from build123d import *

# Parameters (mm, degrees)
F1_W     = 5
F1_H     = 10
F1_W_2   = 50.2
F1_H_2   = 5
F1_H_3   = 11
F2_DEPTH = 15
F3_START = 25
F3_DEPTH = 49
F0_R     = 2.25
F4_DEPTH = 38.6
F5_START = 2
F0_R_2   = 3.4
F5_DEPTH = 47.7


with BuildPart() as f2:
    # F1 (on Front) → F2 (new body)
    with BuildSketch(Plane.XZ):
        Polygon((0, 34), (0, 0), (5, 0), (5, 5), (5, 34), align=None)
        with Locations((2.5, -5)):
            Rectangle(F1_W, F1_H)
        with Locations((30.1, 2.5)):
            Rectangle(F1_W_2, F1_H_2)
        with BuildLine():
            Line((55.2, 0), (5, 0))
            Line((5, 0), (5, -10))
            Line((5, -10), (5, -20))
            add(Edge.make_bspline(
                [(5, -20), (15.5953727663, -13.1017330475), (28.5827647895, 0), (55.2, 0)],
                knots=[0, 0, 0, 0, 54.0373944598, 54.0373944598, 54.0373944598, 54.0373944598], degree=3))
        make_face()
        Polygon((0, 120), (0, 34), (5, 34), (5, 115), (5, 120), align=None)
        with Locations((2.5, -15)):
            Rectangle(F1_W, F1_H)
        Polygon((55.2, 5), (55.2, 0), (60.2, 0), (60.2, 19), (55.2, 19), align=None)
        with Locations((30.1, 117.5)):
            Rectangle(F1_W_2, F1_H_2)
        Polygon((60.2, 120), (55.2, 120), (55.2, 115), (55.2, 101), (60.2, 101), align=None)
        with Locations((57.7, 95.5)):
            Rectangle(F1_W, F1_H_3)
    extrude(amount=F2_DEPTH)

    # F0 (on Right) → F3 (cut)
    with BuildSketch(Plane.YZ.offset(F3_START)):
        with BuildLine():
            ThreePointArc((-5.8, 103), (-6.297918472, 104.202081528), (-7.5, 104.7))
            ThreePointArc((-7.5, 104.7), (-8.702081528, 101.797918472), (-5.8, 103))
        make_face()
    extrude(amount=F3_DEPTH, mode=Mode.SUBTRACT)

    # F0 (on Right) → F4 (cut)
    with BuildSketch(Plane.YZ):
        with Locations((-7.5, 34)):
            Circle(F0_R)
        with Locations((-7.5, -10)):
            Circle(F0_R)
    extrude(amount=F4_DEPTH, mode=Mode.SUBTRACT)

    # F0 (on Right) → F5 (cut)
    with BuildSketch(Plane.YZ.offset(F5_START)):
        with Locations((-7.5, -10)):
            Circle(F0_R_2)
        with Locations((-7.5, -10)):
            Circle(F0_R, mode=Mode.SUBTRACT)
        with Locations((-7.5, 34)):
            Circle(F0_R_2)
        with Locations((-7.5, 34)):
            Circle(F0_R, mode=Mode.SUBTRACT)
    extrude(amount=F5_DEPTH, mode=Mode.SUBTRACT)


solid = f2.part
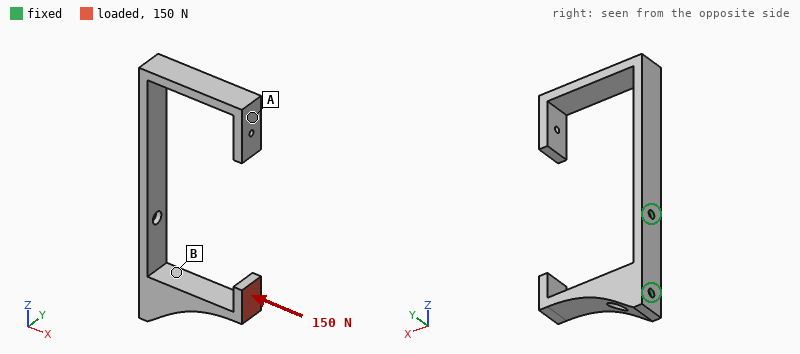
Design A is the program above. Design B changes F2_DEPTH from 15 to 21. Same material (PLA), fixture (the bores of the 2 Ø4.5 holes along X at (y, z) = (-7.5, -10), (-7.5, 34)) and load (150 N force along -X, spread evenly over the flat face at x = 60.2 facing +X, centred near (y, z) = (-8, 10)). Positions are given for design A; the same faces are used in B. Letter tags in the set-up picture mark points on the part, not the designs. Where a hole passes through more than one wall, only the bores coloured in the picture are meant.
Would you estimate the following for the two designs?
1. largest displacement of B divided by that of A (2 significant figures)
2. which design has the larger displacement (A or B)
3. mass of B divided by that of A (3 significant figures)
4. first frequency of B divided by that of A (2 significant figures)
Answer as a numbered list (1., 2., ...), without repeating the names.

1. 0.78
2. A
3. 1.41
4. 0.99
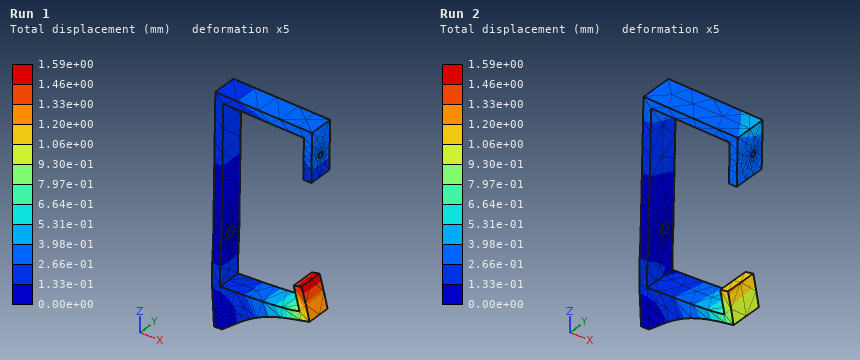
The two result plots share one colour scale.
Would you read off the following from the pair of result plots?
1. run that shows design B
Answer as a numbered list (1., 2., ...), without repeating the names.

1. Run 2
